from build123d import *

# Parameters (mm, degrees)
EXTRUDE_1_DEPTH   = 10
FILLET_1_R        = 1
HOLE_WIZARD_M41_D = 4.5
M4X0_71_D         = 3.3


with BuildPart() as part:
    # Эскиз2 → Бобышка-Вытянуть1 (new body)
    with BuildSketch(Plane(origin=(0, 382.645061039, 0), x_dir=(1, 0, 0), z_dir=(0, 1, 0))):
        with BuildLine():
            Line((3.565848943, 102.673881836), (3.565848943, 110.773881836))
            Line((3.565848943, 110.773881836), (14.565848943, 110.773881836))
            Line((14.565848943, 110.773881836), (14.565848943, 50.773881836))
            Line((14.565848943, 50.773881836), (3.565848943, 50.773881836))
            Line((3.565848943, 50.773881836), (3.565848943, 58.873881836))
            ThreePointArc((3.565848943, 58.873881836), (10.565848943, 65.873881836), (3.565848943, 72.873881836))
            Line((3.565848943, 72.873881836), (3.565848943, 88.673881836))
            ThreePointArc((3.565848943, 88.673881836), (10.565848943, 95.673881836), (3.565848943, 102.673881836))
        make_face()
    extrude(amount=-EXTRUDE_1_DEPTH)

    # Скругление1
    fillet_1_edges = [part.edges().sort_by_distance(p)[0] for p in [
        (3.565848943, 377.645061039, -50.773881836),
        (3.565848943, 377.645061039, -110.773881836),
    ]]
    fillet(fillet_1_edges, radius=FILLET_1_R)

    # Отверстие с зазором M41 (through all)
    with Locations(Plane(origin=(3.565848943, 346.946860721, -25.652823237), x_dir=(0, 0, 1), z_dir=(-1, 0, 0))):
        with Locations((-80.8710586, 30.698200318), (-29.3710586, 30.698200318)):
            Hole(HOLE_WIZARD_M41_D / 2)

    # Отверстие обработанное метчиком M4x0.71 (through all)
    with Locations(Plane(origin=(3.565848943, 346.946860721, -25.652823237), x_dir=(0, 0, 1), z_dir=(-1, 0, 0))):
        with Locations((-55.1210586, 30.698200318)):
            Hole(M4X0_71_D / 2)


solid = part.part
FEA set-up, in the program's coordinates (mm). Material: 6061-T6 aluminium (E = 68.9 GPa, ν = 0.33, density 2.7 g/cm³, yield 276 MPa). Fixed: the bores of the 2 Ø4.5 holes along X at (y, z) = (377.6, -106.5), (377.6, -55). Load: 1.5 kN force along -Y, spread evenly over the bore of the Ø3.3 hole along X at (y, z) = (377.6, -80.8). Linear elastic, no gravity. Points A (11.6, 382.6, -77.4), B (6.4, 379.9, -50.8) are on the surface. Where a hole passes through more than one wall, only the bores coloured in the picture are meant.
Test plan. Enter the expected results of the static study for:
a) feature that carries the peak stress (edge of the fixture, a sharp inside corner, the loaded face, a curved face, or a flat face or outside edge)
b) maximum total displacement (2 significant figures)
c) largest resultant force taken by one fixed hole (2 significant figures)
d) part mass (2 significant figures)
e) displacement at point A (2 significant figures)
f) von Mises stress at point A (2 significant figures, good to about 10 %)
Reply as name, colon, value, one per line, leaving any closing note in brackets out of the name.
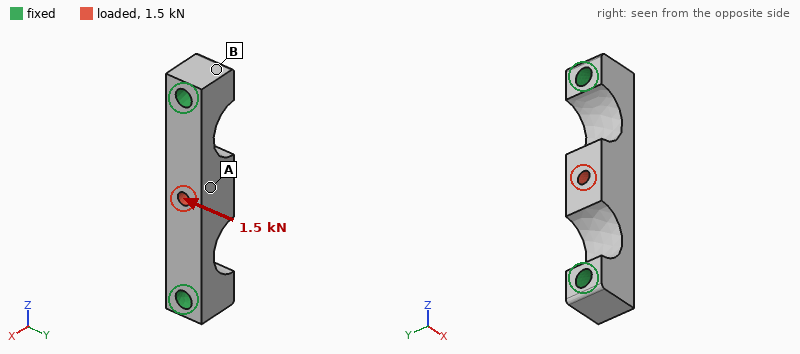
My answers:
feature that carries the peak stress: a curved face
maximum total displacement: 87 µm
largest resultant force taken by one fixed hole: 750 N
part mass: 12 g
displacement at point A: 49 µm
von Mises stress at point A: 58 MPa
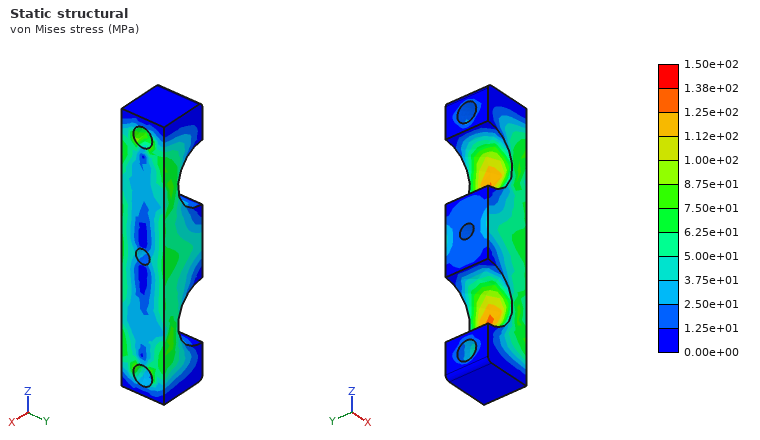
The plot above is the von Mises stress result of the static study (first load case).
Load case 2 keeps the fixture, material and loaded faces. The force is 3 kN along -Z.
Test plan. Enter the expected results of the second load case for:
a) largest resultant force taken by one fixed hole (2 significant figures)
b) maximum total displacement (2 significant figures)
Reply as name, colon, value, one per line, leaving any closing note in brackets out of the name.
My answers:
largest resultant force taken by one fixed hole: 1.5 kN
maximum total displacement: 19 µm
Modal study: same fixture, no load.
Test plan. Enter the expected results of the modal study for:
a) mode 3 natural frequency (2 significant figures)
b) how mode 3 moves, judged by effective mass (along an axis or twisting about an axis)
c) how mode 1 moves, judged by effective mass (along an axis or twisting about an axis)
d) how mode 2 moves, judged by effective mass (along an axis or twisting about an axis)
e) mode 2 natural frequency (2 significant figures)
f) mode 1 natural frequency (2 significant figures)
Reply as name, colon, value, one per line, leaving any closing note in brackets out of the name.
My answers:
mode 3 natural frequency: 20 kHz
how mode 3 moves, judged by effective mass: along Y
how mode 1 moves, judged by effective mass: along Y
how mode 2 moves, judged by effective mass: along X
mode 2 natural frequency: 13 kHz
mode 1 natural frequency: 11 kHz
